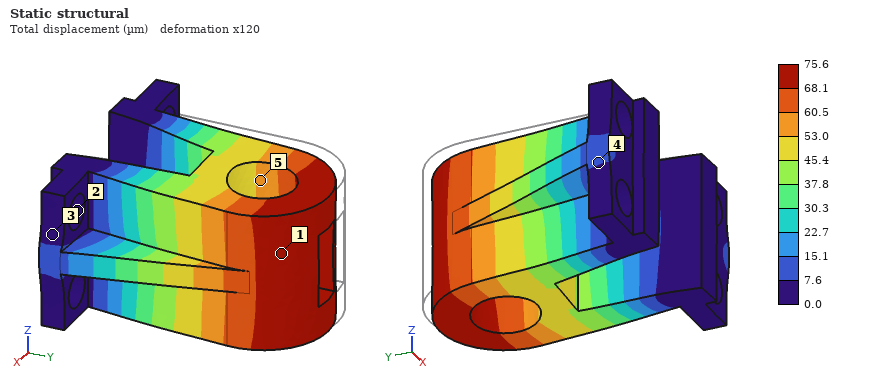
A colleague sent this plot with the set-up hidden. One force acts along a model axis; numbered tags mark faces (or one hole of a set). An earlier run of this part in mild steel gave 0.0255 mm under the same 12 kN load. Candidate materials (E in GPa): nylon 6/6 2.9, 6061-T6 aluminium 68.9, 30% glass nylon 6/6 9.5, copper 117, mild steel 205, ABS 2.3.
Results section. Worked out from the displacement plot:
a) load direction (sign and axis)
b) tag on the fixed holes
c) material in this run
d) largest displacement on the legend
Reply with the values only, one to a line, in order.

+X
2
6061-T6 aluminium
75.6 µm
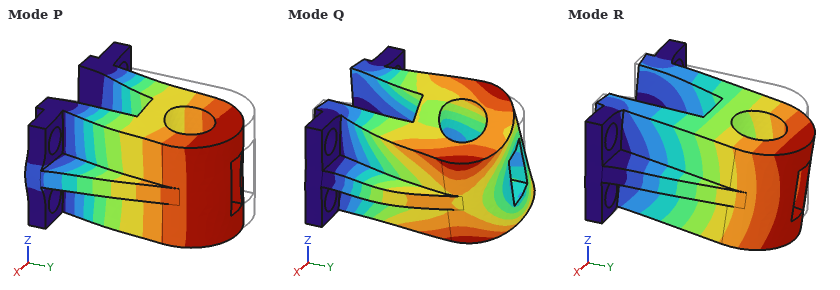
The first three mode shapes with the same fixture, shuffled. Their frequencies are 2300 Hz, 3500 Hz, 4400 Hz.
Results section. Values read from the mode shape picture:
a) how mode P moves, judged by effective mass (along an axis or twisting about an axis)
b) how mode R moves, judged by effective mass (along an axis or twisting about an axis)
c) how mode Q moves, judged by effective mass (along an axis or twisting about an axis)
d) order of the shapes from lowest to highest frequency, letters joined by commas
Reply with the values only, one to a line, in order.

along X
along Z
twisting about Y
R, P, Q
